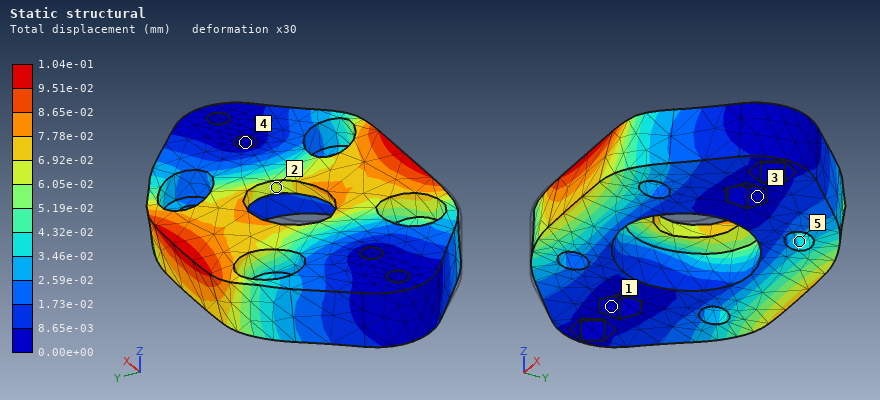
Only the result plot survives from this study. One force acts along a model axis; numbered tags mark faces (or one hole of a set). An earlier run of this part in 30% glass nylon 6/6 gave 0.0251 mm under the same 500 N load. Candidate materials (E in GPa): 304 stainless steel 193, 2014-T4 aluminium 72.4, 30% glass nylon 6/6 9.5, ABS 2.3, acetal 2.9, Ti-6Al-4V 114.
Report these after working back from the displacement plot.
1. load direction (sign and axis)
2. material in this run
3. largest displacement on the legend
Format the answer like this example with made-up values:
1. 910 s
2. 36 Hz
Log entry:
1. +Y
2. ABS
3. 1.04e-01 mm
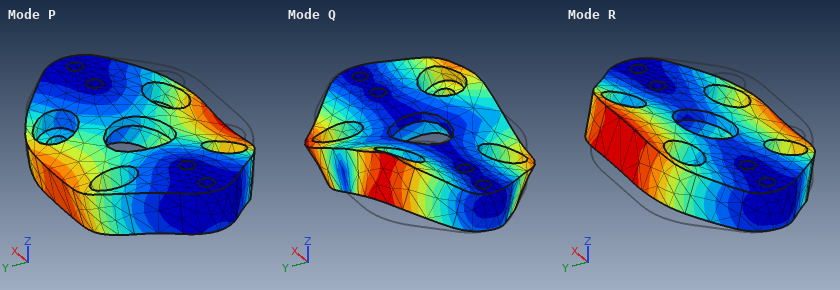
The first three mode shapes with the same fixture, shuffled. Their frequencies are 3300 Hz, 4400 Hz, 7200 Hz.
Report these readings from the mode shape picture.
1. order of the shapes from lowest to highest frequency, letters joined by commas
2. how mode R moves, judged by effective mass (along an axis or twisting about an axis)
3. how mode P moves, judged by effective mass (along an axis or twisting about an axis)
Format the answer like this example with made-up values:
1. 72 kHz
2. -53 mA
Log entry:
1. R, P, Q
2. twisting about X
3. along Z
